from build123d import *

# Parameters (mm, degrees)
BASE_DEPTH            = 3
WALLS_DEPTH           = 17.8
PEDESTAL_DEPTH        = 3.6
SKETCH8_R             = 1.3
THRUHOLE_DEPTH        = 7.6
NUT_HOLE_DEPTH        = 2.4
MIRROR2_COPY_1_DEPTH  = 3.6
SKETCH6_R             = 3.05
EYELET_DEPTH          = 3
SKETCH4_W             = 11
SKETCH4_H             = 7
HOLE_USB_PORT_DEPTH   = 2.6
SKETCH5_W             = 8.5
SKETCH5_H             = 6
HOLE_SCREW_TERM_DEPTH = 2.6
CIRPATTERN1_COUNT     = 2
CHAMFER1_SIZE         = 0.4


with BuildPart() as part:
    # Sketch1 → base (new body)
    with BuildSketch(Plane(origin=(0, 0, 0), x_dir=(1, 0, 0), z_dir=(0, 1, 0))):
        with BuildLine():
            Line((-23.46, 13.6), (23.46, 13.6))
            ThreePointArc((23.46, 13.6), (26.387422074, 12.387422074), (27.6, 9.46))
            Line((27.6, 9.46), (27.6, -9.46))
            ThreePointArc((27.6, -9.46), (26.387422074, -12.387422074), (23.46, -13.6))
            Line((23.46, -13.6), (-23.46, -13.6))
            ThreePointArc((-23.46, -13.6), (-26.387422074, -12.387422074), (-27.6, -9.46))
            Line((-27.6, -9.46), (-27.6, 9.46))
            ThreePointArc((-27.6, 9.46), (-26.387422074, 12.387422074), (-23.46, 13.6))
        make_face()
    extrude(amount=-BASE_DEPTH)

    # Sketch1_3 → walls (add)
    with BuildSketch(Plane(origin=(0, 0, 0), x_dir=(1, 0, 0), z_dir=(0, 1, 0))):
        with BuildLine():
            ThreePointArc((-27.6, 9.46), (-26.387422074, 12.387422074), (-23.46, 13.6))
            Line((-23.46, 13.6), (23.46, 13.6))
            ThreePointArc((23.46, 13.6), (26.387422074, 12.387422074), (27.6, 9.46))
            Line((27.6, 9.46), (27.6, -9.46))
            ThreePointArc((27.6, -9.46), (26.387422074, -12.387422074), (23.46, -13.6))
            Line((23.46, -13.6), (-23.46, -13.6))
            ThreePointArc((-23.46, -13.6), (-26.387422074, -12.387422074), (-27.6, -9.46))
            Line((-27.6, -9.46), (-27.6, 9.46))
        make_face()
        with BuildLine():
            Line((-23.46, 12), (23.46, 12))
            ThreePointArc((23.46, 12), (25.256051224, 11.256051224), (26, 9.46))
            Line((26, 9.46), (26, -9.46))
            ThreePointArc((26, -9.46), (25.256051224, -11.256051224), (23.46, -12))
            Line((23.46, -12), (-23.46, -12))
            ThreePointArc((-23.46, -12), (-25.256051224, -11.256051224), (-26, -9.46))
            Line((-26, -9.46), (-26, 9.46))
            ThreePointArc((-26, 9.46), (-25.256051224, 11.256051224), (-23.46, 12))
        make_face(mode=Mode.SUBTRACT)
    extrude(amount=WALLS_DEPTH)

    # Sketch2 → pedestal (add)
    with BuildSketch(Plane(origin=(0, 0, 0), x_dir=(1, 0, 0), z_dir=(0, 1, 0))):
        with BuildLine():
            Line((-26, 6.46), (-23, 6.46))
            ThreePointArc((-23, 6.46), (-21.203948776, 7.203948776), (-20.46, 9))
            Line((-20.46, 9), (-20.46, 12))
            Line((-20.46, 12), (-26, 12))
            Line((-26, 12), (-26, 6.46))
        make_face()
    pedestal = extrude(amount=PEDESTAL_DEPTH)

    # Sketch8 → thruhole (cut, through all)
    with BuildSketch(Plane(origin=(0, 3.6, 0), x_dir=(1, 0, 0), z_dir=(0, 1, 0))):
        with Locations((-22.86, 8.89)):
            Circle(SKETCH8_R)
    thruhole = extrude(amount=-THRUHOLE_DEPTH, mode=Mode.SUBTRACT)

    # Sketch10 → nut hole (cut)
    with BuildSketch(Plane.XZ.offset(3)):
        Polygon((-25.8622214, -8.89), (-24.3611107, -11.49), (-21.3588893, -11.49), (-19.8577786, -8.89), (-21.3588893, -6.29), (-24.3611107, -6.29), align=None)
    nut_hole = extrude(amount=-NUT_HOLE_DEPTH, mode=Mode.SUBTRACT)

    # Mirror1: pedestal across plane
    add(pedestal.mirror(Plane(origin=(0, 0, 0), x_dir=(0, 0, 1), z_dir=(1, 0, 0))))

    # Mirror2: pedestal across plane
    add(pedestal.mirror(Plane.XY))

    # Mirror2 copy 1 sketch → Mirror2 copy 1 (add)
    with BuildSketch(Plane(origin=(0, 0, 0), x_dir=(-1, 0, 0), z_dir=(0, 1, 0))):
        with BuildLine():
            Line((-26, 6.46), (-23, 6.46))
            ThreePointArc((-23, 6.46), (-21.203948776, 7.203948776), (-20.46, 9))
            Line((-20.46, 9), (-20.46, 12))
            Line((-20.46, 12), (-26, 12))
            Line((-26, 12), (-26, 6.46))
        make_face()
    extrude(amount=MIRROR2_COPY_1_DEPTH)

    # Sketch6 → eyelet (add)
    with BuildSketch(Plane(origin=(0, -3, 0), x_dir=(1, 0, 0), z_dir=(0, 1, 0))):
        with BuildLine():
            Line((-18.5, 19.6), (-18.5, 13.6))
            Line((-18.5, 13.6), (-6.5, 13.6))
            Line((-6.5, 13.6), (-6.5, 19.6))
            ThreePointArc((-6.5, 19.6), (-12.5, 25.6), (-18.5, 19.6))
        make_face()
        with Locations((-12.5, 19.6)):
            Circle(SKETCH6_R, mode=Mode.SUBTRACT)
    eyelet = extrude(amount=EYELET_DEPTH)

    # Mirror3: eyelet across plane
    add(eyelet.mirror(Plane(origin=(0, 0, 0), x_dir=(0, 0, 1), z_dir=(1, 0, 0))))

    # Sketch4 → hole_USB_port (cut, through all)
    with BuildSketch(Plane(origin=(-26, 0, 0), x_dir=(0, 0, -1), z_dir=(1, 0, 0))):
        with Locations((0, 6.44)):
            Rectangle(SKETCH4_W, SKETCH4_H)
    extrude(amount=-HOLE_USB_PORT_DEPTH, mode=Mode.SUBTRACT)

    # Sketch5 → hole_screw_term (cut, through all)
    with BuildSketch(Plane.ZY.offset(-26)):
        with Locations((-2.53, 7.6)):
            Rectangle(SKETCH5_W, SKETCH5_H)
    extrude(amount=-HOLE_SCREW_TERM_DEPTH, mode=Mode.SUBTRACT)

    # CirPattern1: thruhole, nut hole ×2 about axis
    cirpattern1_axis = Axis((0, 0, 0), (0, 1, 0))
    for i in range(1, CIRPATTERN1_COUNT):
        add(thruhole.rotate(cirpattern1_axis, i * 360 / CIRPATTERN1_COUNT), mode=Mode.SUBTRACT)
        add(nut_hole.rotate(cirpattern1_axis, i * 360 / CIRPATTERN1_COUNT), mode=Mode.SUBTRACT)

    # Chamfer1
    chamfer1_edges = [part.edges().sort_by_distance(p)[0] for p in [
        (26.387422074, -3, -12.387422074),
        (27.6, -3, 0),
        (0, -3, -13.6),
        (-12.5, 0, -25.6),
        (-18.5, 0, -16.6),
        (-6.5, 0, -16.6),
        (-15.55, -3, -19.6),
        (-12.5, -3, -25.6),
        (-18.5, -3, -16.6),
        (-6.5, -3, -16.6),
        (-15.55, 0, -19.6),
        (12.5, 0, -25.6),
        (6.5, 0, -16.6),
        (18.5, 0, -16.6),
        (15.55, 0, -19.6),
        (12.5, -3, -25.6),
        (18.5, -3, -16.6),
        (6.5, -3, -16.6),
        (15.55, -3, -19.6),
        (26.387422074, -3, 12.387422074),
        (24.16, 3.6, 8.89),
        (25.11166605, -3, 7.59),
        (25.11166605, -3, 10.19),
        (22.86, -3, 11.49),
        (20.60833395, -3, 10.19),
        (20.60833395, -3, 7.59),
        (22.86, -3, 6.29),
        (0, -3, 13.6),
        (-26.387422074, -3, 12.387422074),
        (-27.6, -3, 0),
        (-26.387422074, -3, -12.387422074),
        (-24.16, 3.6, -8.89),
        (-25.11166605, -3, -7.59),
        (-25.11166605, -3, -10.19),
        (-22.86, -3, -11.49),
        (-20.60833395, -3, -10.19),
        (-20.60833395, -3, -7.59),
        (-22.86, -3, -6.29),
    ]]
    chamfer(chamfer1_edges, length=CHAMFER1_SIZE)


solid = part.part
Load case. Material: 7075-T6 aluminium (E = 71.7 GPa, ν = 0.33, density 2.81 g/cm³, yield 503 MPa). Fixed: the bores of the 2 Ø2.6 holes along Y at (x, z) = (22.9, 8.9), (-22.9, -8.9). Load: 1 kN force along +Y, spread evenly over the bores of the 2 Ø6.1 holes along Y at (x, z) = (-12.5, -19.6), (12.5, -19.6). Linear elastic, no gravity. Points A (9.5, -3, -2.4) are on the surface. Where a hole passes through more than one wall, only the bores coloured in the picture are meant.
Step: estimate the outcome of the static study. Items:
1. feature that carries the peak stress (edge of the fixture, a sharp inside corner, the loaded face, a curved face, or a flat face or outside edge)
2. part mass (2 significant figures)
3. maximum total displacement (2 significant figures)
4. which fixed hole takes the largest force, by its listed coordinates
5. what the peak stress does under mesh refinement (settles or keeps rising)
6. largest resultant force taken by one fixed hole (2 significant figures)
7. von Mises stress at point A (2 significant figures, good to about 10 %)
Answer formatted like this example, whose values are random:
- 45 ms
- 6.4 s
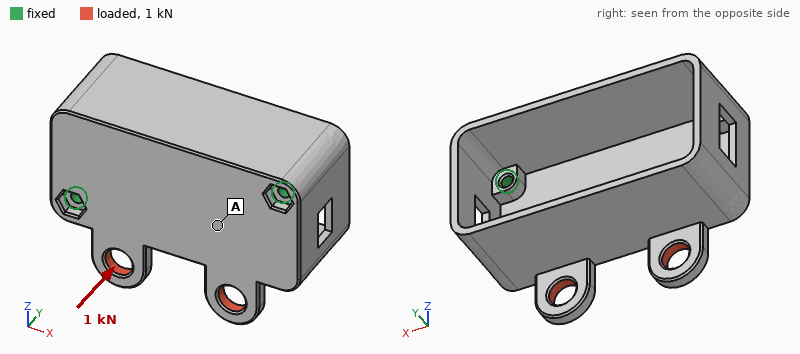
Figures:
- edge of the fixture
- 26 g
- 0.45 mm
- (-22.9, -8.9)
- keeps rising
- 830 N
- 41 MPa
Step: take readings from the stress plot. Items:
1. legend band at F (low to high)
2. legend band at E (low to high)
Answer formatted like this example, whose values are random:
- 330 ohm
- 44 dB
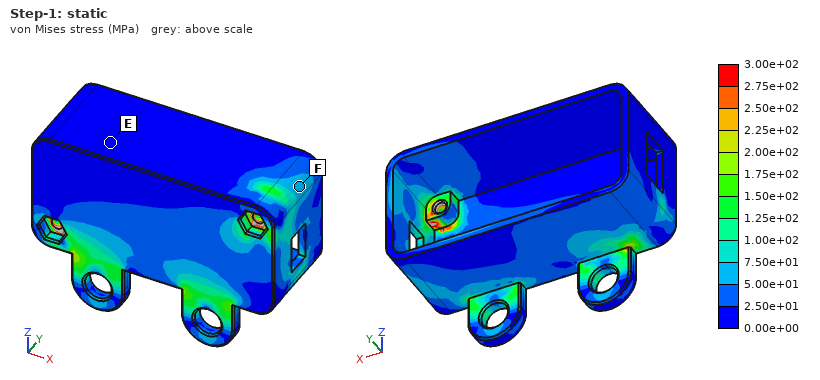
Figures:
- 5.00e+01 to 7.50e+01 MPa
- 0.00e+00 to 2.50e+01 MPa
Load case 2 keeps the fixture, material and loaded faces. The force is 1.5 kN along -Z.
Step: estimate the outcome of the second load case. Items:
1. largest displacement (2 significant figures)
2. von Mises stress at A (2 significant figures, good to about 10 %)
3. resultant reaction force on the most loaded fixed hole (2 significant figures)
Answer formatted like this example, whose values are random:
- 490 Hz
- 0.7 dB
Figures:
- 39 µm
- 10 MPa
- 760 N
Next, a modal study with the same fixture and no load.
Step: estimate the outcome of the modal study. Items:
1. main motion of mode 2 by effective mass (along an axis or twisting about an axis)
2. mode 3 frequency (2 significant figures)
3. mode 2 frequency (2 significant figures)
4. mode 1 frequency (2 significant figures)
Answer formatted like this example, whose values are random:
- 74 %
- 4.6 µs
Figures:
- along Y
- 5100 Hz
- 4300 Hz
- 3500 Hz
